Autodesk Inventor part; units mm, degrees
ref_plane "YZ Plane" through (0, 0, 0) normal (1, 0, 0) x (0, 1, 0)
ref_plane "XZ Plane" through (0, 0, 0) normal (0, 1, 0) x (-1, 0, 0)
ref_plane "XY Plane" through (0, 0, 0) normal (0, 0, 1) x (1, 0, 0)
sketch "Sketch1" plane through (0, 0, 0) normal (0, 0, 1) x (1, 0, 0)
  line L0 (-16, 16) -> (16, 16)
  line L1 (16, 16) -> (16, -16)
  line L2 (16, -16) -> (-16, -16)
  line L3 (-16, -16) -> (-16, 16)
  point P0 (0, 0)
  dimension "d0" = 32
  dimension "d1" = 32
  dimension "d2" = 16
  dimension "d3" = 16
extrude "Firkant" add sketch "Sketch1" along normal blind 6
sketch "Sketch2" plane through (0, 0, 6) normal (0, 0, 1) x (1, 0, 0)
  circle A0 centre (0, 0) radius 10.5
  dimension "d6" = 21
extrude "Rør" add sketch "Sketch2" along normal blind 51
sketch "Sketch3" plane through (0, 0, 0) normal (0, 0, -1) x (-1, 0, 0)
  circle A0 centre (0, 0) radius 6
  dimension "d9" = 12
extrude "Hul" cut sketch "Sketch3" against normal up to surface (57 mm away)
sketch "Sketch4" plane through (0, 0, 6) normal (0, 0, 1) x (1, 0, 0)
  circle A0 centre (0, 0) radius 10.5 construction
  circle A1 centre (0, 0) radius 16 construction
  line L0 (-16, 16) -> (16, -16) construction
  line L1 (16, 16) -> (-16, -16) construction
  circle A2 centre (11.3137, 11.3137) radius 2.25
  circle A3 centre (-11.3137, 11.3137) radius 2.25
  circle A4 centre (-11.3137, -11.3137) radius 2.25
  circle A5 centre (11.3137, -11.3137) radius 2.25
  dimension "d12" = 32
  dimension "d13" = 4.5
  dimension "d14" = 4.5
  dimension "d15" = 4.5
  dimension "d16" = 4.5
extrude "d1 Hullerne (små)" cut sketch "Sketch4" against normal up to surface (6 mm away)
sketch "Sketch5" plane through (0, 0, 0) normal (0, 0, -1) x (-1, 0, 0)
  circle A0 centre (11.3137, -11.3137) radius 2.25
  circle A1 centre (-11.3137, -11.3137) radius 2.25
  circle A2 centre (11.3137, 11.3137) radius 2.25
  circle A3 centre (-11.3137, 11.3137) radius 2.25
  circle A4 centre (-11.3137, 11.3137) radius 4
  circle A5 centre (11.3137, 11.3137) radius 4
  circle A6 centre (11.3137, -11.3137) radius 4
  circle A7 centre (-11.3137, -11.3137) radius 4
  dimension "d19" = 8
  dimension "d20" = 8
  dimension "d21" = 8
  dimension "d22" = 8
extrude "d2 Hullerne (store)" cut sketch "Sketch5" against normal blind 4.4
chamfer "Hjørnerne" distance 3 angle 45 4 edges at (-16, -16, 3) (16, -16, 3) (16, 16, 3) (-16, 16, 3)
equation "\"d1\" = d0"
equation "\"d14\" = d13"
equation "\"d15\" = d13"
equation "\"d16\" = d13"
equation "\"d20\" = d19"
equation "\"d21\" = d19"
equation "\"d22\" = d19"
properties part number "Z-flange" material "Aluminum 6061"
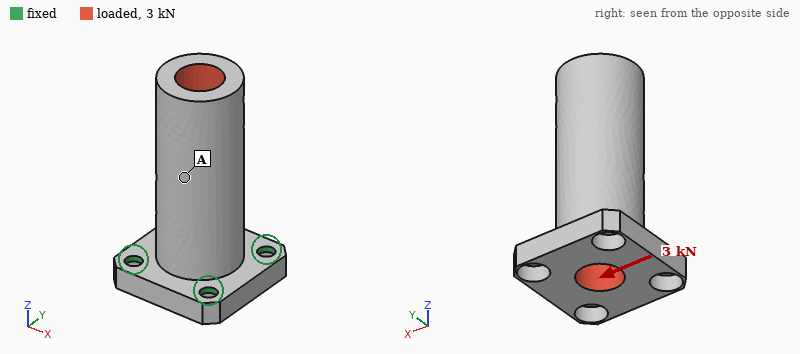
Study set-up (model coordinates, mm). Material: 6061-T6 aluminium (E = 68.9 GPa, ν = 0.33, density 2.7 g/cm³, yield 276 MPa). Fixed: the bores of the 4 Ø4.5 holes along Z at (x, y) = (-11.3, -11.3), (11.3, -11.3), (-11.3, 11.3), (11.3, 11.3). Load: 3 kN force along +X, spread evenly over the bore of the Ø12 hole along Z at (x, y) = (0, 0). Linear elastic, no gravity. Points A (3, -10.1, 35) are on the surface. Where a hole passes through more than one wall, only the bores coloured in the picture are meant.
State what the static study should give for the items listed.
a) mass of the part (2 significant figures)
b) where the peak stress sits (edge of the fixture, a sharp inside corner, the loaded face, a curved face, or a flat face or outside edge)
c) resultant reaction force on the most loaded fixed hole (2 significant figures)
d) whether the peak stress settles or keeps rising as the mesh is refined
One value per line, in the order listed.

44 g
edge of the fixture
1.8 kN
keeps rising
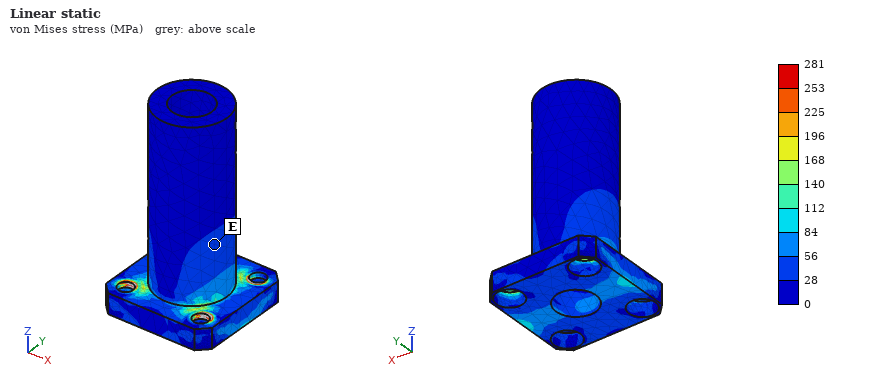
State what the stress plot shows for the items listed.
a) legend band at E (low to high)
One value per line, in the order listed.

28 to 56 MPa
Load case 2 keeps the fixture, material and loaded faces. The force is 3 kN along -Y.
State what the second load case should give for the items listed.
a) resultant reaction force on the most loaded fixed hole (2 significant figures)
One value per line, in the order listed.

1.8 kN
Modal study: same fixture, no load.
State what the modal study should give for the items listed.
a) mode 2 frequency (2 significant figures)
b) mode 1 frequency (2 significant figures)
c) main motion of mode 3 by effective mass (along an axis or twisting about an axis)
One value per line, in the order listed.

3600 Hz
3600 Hz
along Z
